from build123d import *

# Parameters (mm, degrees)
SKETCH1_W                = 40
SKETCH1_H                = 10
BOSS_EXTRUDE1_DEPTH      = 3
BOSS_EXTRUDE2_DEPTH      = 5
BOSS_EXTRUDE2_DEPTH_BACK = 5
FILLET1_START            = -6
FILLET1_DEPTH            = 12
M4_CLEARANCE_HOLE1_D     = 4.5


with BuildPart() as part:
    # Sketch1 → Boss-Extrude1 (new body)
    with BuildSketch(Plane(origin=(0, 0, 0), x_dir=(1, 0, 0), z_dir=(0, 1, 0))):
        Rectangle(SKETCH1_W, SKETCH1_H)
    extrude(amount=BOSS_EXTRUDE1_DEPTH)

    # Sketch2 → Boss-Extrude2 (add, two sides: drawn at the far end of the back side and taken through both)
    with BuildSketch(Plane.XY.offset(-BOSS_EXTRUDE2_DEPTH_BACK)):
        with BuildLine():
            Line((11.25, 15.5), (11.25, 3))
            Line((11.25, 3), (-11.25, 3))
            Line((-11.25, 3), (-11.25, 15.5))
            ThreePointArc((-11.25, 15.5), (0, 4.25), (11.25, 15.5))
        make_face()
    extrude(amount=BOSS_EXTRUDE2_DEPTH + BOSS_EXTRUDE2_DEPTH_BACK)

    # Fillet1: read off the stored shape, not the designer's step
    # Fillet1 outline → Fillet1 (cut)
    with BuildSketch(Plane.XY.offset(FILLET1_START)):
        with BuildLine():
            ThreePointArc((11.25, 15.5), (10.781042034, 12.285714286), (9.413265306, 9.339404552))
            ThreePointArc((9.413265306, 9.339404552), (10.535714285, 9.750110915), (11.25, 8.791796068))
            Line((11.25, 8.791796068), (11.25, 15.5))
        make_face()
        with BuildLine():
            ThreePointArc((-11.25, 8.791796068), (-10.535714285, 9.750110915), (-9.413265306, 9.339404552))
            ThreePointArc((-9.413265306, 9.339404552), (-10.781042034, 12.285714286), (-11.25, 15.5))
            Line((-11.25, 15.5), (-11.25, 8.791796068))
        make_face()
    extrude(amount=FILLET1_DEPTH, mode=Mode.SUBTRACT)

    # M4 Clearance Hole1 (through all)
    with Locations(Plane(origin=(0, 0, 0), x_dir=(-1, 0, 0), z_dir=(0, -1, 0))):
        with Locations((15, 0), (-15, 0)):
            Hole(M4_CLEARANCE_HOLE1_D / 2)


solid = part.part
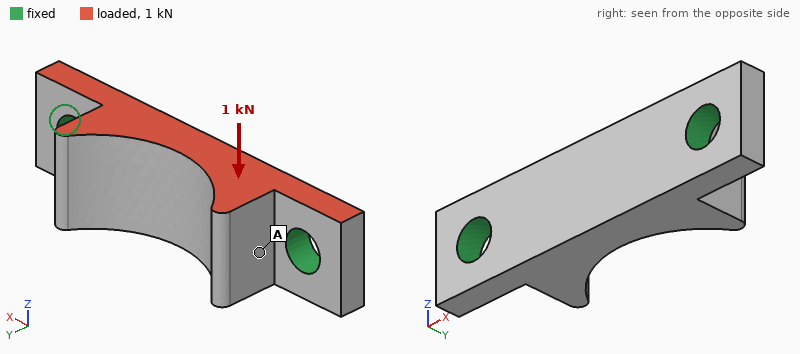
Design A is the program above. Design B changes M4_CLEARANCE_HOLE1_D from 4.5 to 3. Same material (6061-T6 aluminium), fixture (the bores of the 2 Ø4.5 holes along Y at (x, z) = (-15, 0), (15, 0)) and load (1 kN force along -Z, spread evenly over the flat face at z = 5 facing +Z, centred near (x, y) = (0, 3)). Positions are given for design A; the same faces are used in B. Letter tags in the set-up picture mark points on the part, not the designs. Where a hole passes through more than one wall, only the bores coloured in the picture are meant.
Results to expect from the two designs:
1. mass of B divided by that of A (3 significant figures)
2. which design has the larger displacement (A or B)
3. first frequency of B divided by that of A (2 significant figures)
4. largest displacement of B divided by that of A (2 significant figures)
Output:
1.03
B
0.89
1.5
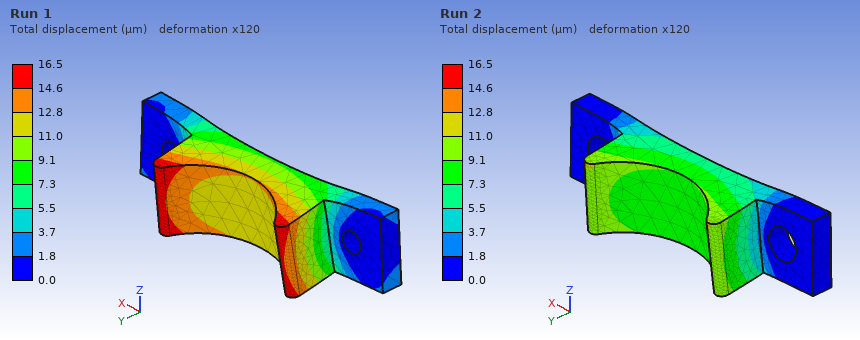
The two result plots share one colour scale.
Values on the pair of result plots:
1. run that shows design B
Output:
Run 1
